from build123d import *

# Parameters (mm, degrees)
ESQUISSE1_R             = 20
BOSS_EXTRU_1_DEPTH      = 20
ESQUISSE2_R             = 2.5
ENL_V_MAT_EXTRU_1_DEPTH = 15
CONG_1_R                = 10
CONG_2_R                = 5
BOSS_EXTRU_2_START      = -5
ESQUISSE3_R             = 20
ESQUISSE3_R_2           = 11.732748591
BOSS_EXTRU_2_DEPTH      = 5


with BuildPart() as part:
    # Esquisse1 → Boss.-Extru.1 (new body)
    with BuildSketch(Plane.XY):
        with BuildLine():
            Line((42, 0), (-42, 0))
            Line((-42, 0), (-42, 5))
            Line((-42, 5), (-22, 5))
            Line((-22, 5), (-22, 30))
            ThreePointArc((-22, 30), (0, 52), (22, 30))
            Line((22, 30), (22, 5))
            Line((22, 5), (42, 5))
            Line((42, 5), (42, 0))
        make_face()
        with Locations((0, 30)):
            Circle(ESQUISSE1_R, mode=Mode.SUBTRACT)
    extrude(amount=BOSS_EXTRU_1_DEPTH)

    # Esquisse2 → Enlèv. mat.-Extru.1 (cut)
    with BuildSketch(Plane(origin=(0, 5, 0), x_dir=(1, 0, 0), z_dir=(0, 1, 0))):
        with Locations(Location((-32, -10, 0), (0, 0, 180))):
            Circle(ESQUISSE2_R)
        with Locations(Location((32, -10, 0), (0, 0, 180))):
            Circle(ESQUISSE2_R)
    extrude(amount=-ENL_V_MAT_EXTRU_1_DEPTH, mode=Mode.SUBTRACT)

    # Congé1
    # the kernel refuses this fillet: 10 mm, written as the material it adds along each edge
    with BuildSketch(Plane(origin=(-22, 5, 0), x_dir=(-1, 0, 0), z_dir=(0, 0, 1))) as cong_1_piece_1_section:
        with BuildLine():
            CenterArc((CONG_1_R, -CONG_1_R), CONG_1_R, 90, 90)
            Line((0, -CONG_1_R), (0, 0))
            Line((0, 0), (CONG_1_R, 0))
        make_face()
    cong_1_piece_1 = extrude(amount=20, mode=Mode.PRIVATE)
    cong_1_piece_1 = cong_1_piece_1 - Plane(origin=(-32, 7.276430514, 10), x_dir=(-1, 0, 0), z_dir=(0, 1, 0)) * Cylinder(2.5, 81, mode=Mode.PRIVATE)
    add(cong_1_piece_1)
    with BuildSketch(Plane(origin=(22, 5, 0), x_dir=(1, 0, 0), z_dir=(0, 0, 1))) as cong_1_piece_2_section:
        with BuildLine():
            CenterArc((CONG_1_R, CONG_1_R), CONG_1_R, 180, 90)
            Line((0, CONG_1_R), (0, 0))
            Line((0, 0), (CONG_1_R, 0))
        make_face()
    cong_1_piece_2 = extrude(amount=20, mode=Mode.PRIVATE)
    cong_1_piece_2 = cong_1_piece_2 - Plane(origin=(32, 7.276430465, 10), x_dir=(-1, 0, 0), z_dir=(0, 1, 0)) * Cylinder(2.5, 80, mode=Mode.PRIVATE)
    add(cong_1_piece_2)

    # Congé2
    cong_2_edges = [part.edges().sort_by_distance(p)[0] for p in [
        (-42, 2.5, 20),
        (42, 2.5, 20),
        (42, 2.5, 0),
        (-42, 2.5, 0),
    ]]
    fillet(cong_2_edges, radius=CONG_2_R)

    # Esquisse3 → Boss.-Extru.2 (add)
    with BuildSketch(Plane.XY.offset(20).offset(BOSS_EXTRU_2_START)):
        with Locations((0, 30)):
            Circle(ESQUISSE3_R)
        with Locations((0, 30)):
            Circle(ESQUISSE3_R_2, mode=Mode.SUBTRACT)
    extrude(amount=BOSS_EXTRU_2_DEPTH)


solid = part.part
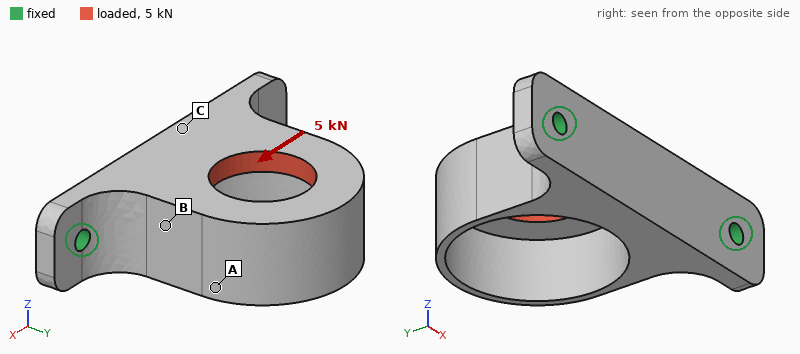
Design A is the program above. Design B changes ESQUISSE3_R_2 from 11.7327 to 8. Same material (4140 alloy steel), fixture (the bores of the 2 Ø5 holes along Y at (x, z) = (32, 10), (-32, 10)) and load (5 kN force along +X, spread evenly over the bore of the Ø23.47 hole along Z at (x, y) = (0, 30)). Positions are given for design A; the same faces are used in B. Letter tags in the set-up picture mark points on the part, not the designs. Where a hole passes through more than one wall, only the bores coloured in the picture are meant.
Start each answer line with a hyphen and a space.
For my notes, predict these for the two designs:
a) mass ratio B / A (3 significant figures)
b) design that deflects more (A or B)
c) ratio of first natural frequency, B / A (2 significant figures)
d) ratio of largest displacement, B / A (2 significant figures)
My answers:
- 1.05
- A
- 0.96
- 0.74
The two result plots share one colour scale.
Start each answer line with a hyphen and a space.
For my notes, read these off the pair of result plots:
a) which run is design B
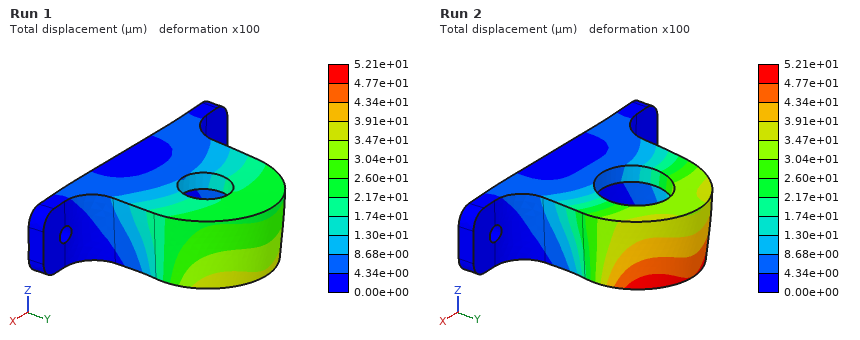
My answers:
- Run 1
